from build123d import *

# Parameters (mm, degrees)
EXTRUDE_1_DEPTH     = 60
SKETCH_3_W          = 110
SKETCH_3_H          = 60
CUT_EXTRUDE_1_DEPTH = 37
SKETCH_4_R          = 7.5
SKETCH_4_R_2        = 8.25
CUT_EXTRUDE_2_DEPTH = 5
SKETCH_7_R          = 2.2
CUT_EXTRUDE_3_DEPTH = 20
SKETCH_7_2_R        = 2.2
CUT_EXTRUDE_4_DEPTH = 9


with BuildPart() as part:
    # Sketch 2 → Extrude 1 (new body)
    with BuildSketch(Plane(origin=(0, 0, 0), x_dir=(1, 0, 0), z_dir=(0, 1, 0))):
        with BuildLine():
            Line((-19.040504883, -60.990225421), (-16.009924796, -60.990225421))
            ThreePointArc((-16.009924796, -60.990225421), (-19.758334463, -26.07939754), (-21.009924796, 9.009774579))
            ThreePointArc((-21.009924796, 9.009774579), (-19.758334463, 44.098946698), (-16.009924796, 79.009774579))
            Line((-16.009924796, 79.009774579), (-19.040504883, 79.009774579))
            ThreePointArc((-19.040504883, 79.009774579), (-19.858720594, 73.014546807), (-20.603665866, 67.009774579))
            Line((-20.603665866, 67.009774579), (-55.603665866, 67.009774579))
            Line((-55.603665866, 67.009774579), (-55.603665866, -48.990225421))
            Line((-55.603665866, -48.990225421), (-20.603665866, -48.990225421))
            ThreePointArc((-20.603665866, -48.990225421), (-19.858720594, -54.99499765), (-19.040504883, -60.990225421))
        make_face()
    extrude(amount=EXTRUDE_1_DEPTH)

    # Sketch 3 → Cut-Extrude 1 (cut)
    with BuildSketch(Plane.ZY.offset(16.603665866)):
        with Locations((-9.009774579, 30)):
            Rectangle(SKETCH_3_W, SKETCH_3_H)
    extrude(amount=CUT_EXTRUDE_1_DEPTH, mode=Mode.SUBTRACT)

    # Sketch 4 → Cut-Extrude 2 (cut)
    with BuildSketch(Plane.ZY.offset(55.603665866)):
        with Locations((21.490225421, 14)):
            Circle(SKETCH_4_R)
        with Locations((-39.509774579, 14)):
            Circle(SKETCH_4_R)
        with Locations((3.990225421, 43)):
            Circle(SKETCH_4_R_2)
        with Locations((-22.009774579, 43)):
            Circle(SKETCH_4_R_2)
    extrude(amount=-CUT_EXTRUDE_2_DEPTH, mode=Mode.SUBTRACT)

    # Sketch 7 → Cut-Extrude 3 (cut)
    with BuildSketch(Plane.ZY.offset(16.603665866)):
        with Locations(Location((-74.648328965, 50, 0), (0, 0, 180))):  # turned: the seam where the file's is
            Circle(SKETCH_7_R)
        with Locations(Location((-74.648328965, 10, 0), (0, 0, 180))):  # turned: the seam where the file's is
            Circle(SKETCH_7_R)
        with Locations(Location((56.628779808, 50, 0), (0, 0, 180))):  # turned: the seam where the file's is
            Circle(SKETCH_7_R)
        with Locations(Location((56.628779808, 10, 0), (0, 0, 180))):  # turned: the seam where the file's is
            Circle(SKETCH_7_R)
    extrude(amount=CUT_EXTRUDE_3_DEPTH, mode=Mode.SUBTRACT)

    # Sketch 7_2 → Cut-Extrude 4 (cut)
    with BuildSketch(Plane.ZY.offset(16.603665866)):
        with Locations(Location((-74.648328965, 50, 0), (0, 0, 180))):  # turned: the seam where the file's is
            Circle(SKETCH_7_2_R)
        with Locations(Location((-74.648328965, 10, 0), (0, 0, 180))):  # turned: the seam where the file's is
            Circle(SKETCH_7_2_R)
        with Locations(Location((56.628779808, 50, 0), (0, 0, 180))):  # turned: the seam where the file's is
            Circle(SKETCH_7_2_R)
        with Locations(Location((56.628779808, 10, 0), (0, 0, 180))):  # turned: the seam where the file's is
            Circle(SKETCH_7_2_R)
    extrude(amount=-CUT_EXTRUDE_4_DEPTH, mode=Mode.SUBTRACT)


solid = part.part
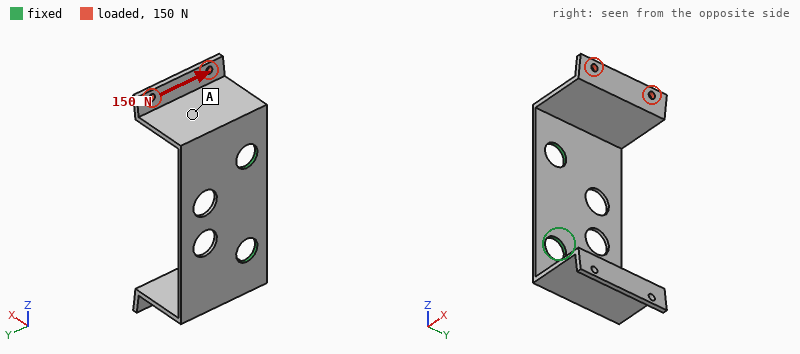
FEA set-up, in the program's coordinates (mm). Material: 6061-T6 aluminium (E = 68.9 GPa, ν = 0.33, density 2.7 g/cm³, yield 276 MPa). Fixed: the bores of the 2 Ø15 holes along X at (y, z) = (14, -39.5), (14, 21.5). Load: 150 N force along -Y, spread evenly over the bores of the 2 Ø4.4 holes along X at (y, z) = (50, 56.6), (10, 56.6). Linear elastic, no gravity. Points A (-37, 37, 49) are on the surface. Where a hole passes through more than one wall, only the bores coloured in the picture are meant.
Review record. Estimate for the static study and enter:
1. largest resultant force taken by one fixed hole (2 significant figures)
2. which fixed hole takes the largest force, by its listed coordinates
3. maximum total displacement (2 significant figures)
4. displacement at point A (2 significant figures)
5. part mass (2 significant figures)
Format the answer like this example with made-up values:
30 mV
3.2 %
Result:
190 N
(14, 21.5)
1.1 mm
0.52 mm
79 g
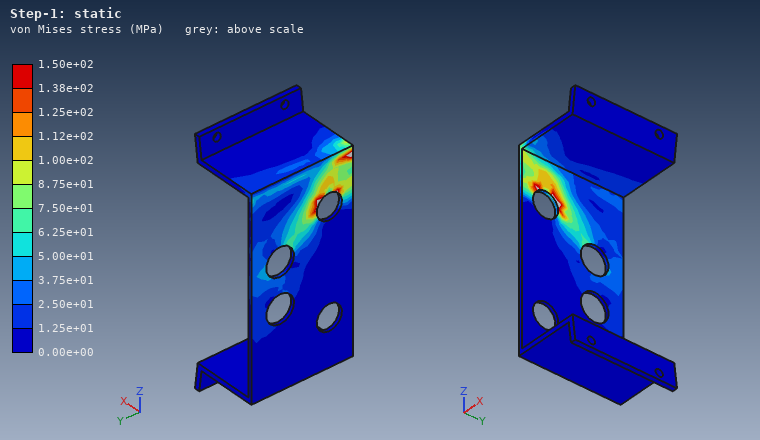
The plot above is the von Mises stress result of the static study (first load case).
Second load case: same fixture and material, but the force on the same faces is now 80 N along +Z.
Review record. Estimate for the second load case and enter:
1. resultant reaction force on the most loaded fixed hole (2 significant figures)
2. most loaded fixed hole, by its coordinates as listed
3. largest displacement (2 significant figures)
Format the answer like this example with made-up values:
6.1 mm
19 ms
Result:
66 N
(14, 21.5)
1.3 mm
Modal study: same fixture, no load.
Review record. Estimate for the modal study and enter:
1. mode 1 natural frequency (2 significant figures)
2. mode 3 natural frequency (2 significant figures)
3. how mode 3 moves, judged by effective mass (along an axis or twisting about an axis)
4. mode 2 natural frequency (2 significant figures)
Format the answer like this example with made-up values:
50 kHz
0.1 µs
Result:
360 Hz
550 Hz
along Y
360 Hz
